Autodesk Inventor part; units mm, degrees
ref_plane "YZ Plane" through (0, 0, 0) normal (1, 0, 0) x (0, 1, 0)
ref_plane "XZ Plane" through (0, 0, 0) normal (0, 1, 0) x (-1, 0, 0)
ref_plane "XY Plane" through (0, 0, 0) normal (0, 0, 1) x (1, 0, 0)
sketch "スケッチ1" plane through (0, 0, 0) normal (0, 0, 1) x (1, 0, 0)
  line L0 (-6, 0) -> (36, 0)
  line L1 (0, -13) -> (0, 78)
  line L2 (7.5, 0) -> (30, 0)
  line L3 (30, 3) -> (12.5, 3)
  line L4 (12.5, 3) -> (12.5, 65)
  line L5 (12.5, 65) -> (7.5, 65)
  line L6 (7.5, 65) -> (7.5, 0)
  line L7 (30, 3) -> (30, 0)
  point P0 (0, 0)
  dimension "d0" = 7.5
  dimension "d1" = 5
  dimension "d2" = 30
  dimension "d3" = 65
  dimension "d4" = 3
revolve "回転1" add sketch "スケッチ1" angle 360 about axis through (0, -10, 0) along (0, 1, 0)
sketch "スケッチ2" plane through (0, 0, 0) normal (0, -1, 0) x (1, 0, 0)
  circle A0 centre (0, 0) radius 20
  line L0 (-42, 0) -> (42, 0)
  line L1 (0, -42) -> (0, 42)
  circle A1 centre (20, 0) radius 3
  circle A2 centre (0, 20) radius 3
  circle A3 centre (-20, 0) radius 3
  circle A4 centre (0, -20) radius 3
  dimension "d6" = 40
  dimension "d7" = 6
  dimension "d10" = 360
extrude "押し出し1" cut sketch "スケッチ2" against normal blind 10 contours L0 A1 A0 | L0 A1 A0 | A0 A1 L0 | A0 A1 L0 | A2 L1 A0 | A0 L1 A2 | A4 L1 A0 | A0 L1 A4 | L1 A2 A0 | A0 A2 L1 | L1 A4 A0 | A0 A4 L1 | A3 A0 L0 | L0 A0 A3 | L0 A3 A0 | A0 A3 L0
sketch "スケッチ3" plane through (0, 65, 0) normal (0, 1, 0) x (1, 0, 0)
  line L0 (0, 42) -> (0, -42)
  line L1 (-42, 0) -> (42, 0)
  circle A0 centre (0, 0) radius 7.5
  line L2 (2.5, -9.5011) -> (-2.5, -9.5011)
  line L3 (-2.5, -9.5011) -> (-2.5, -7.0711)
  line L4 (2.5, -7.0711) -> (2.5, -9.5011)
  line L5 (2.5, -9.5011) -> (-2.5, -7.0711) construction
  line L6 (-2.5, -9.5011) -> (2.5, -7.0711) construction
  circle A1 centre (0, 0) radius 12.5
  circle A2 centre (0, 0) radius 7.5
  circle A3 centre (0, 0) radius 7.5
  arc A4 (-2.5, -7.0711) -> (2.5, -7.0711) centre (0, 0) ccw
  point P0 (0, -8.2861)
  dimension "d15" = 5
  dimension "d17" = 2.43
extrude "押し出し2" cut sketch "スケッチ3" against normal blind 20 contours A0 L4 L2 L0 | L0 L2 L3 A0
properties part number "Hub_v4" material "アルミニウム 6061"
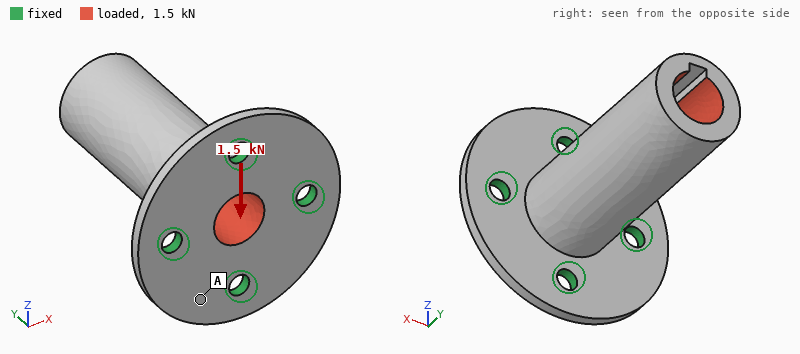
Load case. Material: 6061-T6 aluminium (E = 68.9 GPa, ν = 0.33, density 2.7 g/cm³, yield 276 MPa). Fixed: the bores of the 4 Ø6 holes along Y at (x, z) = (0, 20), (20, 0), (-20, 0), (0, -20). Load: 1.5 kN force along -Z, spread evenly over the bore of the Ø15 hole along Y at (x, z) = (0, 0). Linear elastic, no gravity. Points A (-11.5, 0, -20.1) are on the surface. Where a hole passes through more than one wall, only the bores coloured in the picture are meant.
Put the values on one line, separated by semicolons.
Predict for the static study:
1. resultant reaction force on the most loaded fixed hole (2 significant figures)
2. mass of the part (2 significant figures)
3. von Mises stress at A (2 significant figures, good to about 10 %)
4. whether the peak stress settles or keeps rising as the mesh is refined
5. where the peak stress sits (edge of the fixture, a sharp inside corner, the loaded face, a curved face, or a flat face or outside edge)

1.5 kN; 73 g; 17 MPa; keeps rising; edge of the fixture
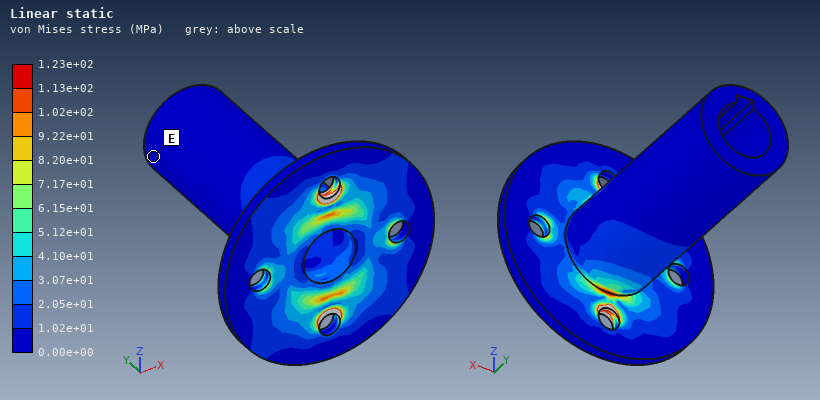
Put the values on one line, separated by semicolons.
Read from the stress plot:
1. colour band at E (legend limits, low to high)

0.00e+00 to 1.02e+01 MPa
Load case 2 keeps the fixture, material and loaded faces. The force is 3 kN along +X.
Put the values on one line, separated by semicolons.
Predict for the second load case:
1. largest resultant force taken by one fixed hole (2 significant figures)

3.0 kN
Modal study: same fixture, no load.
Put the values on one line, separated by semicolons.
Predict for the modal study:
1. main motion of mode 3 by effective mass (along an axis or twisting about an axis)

along Y
